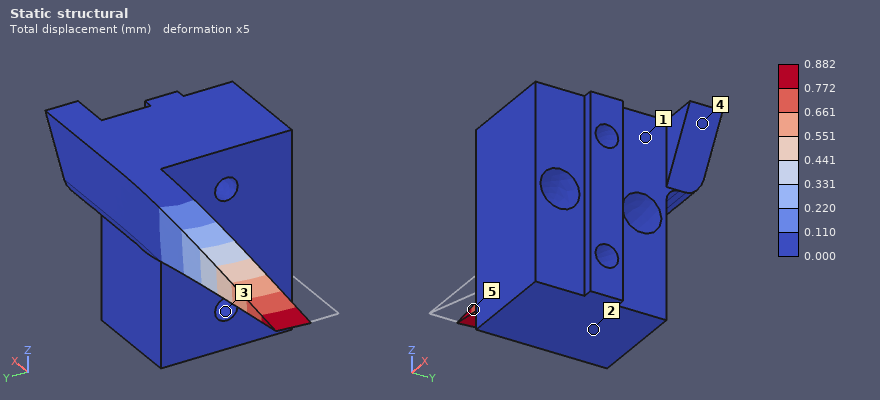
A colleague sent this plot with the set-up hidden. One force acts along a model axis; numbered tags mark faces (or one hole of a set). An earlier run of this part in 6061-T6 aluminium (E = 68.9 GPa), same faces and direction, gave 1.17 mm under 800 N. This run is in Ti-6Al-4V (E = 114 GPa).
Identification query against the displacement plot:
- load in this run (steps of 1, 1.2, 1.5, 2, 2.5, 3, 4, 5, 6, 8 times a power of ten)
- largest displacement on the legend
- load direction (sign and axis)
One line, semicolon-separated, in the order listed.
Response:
1 kN; 0.882 mm; +Y
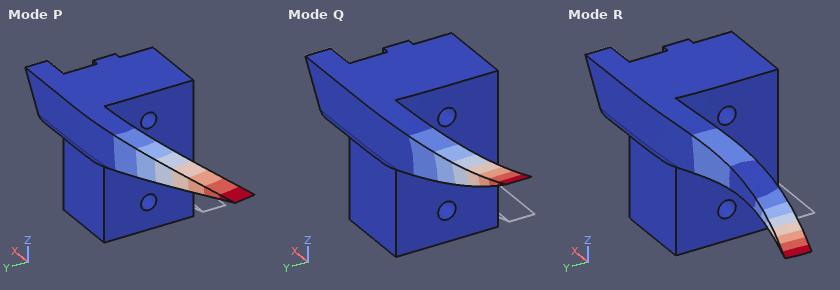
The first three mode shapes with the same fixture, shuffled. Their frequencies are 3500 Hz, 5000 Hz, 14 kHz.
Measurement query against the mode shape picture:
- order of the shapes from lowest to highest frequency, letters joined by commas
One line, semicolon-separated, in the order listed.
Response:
P, Q, R
